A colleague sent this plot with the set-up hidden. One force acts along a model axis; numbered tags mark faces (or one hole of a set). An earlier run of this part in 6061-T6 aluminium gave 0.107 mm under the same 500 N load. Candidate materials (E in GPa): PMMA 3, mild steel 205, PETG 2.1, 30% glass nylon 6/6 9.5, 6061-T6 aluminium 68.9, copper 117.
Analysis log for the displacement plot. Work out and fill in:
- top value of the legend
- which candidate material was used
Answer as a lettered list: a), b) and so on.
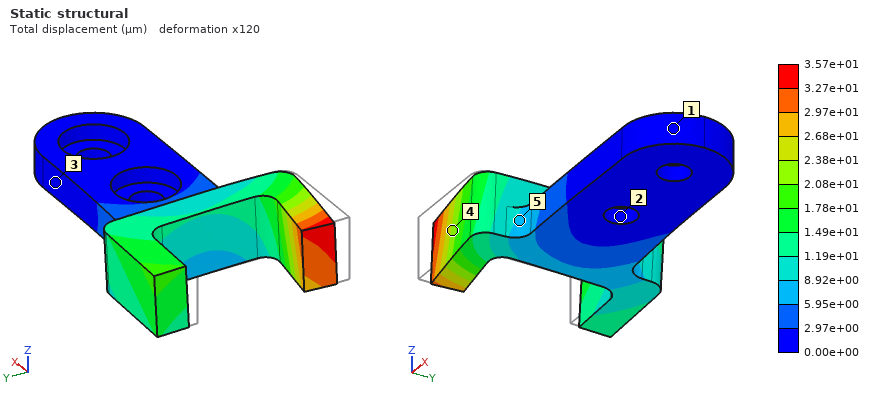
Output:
a) 3.57e+01 µm
b) mild steel
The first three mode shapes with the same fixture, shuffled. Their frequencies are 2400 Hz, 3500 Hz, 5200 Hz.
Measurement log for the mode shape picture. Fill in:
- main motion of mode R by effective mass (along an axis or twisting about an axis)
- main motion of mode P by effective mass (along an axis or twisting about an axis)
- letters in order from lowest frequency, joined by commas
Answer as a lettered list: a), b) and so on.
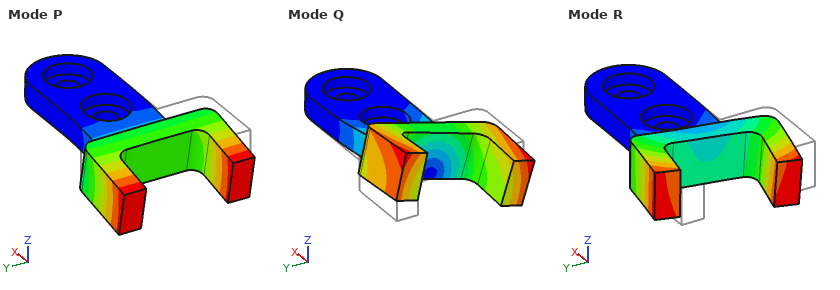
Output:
a) along Y
b) along Z
c) P, Q, R
